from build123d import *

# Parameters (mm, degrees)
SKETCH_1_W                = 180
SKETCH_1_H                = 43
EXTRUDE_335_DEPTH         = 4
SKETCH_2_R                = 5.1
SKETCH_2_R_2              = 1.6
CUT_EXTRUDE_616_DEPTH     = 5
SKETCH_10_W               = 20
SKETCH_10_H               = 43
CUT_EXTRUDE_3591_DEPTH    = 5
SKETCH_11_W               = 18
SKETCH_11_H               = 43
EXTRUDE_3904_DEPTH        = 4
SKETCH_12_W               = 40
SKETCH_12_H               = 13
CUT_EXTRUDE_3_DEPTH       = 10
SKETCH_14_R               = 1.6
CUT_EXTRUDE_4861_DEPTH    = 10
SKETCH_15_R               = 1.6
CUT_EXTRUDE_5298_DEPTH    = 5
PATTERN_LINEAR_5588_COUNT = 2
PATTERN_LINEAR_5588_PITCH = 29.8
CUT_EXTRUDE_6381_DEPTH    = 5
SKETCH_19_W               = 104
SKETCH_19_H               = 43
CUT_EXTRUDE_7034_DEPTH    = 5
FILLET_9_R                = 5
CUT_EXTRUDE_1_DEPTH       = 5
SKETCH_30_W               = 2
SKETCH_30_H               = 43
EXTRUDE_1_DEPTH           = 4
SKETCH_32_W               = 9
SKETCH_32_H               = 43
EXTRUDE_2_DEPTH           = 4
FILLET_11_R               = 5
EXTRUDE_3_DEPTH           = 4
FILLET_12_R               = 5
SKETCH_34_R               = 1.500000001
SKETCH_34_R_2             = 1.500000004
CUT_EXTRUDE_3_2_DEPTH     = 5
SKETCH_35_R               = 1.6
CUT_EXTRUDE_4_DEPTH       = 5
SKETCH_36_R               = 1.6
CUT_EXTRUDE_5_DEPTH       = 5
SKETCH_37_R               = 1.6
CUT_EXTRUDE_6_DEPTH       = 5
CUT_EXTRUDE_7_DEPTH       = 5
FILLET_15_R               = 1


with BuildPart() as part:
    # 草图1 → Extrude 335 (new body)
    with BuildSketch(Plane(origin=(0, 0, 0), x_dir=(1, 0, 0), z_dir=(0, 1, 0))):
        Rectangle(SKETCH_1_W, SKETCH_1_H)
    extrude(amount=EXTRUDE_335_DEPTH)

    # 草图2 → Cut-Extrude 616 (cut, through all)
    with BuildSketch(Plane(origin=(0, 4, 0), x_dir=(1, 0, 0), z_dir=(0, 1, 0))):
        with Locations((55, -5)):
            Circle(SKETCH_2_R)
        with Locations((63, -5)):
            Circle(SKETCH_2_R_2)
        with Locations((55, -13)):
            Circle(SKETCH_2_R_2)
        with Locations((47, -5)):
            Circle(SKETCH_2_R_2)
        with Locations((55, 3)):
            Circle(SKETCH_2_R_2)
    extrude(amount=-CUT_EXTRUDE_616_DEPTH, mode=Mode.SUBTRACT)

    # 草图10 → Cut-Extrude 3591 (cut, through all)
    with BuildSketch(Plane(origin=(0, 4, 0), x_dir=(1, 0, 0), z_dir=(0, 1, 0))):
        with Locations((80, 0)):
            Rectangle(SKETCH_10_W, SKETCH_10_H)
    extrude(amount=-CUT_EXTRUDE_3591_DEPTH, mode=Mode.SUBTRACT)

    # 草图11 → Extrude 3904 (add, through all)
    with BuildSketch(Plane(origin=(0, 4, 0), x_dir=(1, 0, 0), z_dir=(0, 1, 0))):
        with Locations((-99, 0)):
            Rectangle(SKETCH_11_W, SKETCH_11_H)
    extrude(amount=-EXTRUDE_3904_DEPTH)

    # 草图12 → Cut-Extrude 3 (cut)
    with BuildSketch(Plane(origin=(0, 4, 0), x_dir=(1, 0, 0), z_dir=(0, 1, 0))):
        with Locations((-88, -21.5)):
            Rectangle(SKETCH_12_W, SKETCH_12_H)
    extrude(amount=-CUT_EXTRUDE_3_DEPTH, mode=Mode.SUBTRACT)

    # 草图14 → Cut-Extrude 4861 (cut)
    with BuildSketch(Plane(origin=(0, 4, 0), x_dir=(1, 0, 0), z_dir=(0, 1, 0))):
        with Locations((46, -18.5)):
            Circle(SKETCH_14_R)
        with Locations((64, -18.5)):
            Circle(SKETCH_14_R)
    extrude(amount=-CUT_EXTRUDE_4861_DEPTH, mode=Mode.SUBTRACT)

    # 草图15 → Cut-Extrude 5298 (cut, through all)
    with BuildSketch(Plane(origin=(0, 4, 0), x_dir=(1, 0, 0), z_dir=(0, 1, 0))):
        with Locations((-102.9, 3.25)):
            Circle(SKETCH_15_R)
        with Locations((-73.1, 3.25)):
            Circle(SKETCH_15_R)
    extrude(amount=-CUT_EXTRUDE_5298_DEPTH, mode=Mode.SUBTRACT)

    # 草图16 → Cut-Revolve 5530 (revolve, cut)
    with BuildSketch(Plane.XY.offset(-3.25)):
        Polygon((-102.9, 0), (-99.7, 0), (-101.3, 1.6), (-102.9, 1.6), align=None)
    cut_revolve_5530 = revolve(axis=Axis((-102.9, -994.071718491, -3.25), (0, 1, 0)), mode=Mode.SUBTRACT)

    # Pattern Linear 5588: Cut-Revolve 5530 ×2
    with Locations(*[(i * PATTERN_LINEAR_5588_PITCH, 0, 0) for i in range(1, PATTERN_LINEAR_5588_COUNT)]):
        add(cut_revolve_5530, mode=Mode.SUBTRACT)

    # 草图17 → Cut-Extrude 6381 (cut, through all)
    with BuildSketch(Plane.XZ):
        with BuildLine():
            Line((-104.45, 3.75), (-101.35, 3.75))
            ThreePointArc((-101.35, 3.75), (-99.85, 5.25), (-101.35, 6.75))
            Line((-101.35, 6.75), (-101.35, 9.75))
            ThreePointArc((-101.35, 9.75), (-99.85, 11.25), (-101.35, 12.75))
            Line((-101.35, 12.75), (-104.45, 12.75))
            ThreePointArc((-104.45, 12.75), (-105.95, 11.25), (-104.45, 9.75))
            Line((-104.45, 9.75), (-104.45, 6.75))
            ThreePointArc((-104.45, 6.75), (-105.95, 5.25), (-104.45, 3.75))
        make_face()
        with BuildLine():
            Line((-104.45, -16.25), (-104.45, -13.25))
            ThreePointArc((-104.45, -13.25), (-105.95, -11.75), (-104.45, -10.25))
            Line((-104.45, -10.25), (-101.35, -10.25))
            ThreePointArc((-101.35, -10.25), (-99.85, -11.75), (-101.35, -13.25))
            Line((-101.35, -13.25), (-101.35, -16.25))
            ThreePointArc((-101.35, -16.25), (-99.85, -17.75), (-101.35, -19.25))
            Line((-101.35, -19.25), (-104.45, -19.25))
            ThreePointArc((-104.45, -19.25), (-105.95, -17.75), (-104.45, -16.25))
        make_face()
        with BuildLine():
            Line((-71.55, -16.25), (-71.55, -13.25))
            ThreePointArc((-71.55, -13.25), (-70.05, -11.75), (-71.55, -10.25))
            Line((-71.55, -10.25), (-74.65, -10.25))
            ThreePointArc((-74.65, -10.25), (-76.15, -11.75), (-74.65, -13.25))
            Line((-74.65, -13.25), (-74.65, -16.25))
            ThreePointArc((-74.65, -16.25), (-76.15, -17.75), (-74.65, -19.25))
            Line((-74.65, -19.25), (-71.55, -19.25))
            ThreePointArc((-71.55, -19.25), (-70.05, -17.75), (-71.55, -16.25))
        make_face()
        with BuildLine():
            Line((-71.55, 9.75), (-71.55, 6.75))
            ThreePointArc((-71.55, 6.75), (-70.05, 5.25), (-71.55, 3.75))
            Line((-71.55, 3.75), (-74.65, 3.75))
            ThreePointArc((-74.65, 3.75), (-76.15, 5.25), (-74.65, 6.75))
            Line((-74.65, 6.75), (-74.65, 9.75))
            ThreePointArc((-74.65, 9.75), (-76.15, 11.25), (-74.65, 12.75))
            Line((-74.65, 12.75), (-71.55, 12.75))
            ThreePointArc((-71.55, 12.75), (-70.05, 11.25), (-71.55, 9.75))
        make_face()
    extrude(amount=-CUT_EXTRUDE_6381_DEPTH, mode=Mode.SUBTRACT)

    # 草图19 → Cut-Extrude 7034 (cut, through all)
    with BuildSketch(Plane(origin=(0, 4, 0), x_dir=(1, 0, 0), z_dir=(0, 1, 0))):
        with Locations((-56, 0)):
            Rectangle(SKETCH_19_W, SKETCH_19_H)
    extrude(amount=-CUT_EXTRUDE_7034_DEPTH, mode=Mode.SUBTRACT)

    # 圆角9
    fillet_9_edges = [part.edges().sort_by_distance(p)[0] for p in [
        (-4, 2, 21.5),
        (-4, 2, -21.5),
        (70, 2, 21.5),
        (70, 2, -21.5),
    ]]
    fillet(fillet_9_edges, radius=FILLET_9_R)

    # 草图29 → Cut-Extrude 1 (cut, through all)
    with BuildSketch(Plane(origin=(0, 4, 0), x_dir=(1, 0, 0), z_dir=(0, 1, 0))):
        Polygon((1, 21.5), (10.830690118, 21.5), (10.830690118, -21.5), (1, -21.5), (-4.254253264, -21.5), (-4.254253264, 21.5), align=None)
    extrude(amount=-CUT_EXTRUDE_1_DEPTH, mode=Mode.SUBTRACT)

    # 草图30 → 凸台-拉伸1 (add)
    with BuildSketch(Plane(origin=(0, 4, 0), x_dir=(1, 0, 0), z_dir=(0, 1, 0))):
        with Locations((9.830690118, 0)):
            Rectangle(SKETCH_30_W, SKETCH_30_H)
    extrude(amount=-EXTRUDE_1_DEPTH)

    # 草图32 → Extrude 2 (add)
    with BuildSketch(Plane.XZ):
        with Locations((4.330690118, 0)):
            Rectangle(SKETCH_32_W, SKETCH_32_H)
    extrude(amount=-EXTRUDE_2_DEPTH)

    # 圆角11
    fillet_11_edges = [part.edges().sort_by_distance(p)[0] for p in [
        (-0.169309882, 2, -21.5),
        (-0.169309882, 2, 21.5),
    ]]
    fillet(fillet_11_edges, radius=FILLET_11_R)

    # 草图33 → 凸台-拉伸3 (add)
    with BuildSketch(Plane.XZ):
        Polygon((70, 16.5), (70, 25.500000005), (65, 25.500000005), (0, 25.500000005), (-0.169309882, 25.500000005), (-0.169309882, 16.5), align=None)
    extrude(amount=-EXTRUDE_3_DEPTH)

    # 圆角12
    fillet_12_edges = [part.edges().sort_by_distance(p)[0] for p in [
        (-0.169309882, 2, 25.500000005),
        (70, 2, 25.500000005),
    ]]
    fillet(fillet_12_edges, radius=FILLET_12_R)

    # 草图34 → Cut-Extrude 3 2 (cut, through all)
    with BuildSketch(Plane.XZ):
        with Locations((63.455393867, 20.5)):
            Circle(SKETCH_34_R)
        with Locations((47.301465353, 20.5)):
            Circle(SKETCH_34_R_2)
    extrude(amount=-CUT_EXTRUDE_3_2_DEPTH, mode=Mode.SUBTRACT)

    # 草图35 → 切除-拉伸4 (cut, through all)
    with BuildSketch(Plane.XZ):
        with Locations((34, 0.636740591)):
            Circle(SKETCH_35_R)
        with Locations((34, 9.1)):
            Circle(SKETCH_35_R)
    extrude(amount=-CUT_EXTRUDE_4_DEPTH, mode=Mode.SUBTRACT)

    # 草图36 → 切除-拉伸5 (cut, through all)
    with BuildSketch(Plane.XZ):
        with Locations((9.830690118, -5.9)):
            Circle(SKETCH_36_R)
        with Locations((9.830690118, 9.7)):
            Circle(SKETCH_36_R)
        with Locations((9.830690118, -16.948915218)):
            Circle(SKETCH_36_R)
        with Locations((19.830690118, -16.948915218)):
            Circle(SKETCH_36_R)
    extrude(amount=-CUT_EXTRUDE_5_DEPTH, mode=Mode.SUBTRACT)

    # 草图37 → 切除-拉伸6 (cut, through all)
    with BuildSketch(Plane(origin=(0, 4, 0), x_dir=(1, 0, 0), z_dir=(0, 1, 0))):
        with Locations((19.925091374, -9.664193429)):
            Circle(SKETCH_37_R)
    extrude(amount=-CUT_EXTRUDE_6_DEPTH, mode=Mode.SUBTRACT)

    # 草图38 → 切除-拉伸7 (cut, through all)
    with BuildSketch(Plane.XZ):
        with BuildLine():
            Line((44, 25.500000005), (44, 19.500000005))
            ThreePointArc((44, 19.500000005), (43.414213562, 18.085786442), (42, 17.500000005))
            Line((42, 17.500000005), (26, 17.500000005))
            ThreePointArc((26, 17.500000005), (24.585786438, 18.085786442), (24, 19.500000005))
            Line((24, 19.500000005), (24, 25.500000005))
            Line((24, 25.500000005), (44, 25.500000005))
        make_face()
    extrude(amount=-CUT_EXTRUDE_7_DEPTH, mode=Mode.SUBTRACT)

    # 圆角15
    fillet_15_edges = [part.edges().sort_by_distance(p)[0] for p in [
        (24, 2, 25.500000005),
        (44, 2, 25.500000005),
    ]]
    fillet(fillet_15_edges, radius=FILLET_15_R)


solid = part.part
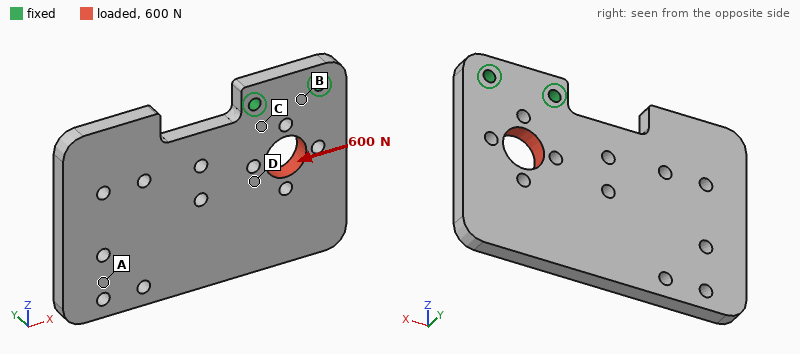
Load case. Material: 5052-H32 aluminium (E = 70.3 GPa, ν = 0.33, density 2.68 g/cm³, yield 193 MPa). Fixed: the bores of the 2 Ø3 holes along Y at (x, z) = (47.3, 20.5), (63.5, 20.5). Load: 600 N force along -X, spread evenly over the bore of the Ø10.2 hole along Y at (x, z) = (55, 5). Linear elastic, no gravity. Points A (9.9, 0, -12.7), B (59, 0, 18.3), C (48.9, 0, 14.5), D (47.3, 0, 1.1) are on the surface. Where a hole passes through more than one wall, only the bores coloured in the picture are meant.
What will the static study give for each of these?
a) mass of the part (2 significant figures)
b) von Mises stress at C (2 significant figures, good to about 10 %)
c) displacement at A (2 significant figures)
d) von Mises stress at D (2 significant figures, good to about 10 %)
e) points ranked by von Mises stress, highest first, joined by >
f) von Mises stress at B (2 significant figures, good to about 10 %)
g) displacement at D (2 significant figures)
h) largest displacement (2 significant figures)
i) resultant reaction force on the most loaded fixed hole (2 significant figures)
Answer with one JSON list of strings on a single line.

["31 g", "16 MPa", "24 µm", "7.0 MPa", "C > B > D > A", "12 MPa", "11 µm", "29 µm", "580 N"]
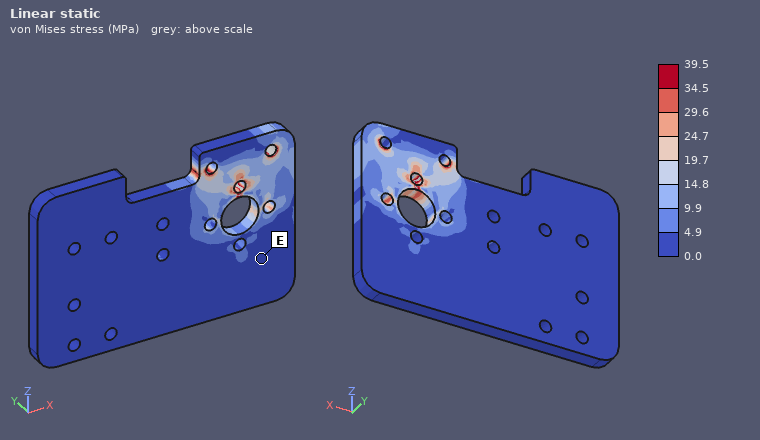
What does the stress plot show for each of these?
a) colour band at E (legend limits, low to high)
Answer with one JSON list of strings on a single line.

["0.0 to 4.9 MPa"]
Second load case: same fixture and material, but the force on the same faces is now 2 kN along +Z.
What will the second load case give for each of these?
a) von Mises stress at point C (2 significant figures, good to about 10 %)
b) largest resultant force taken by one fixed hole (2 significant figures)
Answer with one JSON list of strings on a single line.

["28 MPa", "1.1 kN"]
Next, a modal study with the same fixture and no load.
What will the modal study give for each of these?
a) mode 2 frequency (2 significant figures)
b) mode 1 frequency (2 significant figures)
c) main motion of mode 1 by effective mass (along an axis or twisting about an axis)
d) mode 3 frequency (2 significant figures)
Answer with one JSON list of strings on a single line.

["1400 Hz", "770 Hz", "along Y", "3200 Hz"]
